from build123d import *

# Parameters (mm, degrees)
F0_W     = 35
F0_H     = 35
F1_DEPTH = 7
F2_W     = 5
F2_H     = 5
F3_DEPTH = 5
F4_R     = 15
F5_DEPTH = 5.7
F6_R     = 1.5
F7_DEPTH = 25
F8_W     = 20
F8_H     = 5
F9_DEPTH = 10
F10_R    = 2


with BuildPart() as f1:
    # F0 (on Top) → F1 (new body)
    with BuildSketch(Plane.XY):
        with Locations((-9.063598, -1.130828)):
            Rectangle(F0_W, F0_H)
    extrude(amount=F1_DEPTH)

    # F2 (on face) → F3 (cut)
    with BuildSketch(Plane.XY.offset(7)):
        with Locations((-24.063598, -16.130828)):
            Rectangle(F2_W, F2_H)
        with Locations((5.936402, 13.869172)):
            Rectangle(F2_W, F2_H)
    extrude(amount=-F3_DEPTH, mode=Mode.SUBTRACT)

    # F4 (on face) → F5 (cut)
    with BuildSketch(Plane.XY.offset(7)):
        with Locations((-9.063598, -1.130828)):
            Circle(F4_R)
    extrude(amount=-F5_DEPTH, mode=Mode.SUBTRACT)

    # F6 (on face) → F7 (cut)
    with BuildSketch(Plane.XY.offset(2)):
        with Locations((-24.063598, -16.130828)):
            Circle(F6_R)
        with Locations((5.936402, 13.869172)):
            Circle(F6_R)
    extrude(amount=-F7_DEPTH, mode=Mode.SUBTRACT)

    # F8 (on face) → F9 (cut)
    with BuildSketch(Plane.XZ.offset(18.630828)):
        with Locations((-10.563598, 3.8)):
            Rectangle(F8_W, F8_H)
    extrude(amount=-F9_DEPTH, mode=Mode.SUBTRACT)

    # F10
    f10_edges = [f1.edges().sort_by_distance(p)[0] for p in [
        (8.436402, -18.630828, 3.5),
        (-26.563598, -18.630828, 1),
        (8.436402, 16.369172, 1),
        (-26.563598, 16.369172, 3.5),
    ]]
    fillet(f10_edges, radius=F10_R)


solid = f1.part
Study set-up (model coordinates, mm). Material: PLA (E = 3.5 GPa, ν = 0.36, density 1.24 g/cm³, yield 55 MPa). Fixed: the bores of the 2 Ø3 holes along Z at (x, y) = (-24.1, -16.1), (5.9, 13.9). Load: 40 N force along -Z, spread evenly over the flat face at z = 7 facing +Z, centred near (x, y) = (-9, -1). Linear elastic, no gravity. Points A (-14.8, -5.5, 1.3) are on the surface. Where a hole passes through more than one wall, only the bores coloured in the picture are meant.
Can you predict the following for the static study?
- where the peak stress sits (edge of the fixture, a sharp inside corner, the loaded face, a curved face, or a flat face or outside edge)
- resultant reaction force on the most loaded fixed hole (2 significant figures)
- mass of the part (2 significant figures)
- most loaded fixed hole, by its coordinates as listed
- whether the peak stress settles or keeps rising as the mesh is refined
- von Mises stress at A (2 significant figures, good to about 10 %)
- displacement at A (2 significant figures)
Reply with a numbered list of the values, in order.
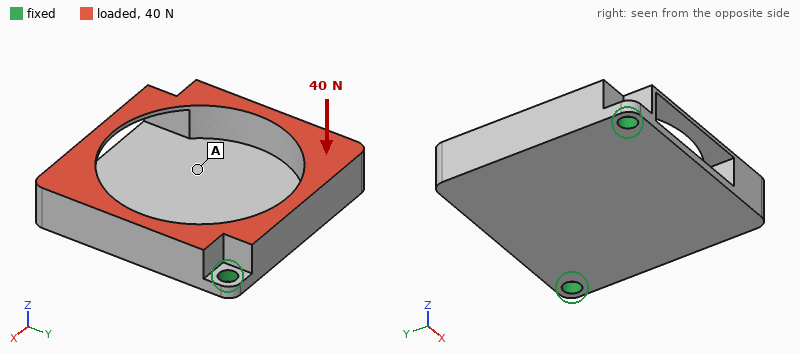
1. edge of the fixture
2. 24 N
3. 4.8 g
4. (5.9, 13.9)
5. keeps rising
6. 3.1 MPa
7. 0.091 mm
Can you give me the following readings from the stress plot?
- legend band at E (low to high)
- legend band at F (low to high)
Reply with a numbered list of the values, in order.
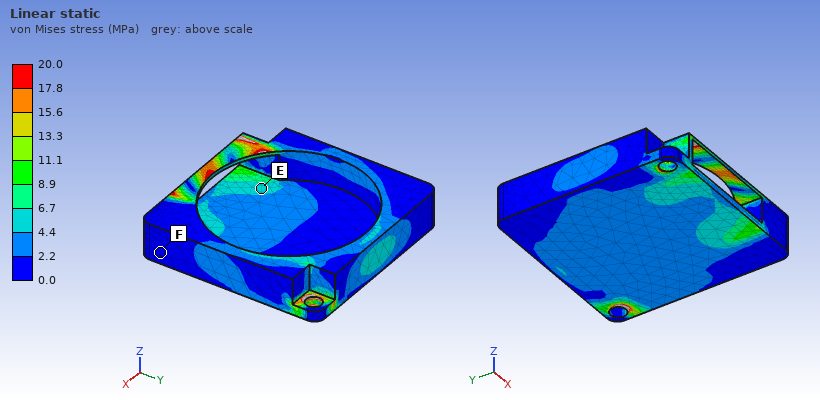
1. 4.4 to 6.7 MPa
2. 0.0 to 2.2 MPa
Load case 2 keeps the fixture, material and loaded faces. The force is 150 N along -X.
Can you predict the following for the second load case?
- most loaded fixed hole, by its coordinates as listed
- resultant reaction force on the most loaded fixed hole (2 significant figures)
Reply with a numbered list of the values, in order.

1. (5.9, 13.9)
2. 84 N
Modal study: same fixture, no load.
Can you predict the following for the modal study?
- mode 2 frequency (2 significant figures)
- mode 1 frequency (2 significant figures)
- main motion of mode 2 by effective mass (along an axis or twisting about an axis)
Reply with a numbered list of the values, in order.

1. 1200 Hz
2. 830 Hz
3. along Z
